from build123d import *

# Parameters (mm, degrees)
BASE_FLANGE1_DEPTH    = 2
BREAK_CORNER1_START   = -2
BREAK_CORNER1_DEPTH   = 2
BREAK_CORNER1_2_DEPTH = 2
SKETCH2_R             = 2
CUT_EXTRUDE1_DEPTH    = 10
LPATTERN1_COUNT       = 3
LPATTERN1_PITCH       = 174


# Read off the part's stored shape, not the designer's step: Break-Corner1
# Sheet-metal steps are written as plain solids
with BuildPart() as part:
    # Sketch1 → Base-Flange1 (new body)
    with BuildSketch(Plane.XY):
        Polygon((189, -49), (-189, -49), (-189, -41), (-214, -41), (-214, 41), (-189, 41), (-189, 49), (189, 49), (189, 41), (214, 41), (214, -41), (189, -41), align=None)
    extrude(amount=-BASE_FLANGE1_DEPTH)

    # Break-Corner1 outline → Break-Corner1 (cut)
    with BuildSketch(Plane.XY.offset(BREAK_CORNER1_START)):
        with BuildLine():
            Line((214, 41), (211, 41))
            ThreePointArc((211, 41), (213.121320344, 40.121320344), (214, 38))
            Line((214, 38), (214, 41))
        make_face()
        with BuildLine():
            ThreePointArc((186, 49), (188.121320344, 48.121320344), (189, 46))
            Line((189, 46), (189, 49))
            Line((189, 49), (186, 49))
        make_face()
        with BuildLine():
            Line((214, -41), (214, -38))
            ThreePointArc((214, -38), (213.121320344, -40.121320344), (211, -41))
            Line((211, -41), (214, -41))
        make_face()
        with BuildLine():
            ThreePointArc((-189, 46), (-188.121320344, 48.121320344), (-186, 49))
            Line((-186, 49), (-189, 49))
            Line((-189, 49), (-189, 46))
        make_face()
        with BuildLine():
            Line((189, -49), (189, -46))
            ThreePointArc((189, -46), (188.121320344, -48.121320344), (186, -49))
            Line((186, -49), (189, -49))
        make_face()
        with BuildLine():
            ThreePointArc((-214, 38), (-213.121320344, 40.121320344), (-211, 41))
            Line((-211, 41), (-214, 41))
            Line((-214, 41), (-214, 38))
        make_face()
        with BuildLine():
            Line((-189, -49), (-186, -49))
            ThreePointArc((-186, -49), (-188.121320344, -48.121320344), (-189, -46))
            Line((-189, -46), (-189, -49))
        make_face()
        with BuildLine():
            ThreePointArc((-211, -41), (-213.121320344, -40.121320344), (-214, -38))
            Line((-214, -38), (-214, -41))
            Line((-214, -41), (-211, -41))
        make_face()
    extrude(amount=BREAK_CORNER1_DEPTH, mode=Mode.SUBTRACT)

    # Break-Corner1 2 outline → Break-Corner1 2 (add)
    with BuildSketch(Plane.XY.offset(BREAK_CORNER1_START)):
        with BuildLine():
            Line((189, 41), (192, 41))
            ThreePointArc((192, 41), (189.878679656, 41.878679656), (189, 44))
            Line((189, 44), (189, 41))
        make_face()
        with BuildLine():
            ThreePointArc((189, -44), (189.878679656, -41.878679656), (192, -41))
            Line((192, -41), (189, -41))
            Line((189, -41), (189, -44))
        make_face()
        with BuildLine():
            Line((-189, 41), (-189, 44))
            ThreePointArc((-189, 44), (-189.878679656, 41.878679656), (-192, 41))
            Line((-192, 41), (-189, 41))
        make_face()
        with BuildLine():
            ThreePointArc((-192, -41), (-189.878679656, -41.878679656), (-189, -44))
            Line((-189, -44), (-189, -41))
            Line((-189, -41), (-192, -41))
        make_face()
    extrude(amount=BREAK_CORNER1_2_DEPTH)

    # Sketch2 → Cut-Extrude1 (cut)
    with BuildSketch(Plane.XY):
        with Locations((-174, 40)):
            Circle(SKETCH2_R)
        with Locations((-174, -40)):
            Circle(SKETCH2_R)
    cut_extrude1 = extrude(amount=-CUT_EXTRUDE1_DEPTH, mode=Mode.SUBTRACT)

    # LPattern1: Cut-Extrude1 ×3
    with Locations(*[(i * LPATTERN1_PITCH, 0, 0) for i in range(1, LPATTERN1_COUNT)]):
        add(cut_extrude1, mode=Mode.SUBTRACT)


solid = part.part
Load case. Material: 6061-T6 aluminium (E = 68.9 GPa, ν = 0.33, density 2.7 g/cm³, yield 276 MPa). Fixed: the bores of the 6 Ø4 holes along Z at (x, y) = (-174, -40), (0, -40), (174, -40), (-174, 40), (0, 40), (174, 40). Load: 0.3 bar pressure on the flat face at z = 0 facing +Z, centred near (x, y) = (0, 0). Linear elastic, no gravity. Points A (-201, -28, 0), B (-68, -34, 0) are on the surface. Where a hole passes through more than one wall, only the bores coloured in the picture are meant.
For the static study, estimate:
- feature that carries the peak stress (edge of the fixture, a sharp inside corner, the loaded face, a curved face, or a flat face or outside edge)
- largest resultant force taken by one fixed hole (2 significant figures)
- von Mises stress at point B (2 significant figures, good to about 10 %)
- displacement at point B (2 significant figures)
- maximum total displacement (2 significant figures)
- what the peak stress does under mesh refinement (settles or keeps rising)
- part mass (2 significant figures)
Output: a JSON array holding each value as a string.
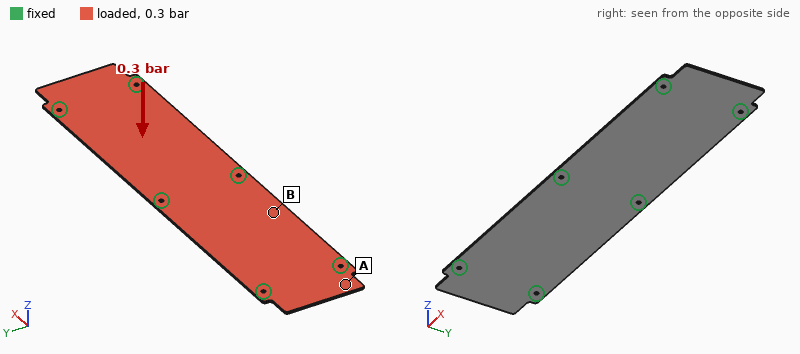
["edge of the fixture", "260 N", "48 MPa", "1.5 mm", "1.7 mm", "keeps rising", "220 g"]
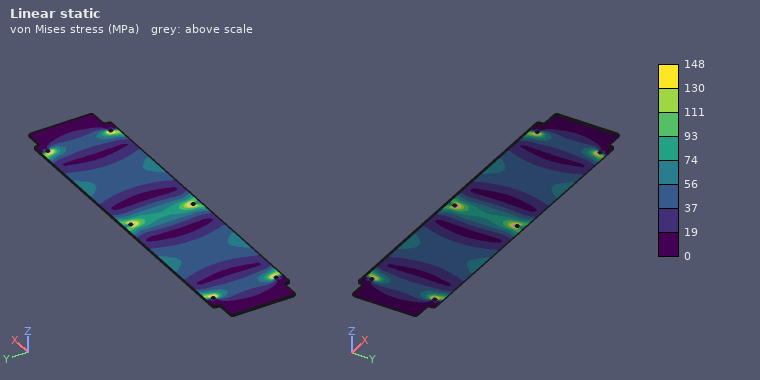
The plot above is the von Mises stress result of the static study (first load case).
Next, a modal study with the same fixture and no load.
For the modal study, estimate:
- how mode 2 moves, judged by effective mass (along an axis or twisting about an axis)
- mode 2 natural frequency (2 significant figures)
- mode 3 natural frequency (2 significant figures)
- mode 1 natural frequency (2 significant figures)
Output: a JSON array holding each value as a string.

["along Z", "330 Hz", "530 Hz", "300 Hz"]
